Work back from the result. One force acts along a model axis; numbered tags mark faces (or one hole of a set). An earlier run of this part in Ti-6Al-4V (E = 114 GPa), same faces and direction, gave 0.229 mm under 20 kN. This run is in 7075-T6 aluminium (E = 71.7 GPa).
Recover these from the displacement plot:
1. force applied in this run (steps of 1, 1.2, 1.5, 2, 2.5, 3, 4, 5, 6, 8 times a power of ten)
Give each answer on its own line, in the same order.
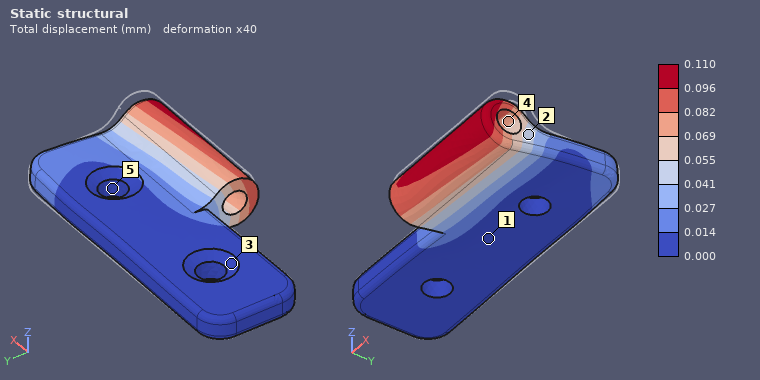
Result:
6 kN
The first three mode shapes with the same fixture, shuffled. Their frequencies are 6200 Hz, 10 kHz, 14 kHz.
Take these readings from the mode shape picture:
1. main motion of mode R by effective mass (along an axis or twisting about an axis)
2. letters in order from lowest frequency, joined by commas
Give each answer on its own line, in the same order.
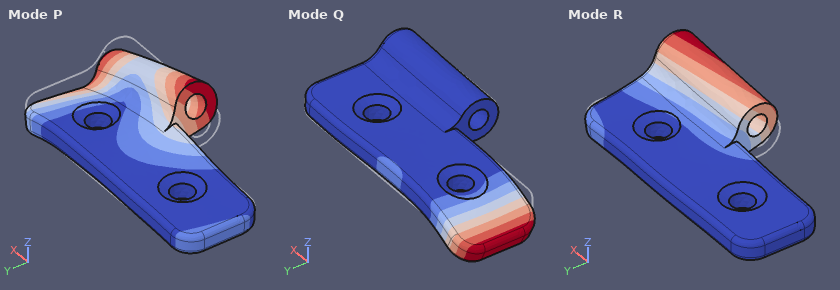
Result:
along Z
R, P, Q
